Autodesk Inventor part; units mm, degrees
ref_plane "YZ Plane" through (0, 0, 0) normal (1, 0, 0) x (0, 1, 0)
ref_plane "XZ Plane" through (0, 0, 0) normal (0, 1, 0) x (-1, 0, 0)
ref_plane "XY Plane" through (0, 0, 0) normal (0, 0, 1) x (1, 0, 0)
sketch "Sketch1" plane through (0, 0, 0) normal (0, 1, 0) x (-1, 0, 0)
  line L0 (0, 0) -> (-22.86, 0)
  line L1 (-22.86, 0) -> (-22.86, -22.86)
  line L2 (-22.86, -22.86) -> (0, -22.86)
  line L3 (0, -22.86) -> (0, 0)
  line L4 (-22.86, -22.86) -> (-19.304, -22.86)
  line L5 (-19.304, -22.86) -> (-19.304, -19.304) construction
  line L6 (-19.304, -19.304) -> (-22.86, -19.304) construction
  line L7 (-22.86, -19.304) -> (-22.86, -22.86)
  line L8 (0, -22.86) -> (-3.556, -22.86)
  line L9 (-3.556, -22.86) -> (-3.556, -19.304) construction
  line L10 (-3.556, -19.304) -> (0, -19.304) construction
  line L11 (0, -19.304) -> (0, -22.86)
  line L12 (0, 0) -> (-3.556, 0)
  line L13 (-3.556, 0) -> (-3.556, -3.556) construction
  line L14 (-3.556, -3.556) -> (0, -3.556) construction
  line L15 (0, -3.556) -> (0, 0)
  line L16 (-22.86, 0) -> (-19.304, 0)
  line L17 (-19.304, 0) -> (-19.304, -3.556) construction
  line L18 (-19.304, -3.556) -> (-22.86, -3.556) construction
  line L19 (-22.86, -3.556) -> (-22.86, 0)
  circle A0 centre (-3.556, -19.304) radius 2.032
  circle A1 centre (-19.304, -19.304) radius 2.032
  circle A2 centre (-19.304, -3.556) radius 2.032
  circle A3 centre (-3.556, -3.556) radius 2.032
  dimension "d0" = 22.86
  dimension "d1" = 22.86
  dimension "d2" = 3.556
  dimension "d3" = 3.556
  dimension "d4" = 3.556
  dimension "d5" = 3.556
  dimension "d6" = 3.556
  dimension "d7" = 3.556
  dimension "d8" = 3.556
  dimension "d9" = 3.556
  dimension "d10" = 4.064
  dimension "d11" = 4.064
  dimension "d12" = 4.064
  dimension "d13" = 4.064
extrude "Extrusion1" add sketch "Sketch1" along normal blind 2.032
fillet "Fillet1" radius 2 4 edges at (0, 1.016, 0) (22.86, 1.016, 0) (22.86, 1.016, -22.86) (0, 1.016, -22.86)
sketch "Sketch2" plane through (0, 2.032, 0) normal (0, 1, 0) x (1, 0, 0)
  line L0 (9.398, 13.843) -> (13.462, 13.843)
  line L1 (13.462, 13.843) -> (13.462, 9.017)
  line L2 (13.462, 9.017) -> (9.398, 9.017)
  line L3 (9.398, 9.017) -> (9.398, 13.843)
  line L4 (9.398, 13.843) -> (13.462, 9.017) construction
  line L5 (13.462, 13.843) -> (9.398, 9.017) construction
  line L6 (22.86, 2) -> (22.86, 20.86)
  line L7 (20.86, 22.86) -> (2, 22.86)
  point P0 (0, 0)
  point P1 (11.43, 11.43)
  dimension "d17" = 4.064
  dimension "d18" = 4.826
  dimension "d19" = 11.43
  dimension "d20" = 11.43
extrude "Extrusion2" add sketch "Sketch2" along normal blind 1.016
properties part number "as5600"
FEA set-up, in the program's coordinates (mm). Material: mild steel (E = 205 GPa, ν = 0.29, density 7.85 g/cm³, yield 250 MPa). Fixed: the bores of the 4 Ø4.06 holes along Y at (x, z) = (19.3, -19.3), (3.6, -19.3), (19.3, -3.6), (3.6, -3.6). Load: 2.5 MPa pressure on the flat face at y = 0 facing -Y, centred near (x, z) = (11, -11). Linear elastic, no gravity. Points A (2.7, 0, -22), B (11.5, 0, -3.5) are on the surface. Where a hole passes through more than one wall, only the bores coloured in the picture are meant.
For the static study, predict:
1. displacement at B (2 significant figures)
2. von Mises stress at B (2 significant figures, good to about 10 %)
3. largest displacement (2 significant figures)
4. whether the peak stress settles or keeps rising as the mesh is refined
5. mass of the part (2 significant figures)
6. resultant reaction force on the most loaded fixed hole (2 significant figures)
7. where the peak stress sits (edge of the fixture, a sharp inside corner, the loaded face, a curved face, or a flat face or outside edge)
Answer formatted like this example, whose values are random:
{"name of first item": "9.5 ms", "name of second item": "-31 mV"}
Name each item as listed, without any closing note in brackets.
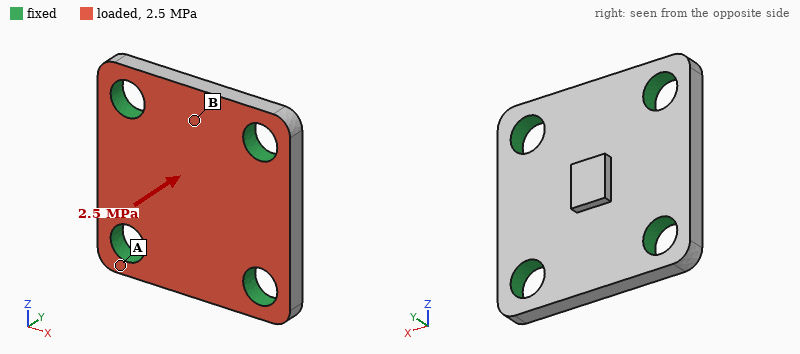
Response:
{"displacement at B": "1.9 µm", "von Mises stress at B": "28 MPa", "largest displacement": "3.3 µm", "whether the peak stress settles or keeps rising as the mesh is refined": "keeps rising", "mass of the part": "7.6 g", "resultant reaction force on the most loaded fixed hole": "290 N", "where the peak stress sits": "edge of the fixture"}
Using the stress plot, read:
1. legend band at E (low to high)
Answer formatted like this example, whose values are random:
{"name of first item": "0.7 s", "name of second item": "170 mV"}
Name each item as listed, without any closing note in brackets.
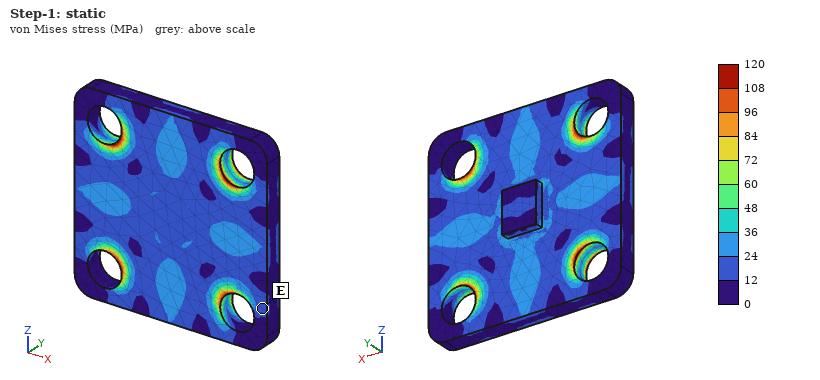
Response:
{"legend band at E": "12 to 24 MPa"}
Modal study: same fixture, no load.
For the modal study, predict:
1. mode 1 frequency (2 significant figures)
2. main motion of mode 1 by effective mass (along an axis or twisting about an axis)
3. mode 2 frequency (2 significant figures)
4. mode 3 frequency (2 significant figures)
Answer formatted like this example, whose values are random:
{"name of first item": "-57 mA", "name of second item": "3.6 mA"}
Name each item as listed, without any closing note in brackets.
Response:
{"mode 1 frequency": "39 kHz", "main motion of mode 1 by effective mass": "along Y", "mode 2 frequency": "59 kHz", "mode 3 frequency": "59 kHz"}
